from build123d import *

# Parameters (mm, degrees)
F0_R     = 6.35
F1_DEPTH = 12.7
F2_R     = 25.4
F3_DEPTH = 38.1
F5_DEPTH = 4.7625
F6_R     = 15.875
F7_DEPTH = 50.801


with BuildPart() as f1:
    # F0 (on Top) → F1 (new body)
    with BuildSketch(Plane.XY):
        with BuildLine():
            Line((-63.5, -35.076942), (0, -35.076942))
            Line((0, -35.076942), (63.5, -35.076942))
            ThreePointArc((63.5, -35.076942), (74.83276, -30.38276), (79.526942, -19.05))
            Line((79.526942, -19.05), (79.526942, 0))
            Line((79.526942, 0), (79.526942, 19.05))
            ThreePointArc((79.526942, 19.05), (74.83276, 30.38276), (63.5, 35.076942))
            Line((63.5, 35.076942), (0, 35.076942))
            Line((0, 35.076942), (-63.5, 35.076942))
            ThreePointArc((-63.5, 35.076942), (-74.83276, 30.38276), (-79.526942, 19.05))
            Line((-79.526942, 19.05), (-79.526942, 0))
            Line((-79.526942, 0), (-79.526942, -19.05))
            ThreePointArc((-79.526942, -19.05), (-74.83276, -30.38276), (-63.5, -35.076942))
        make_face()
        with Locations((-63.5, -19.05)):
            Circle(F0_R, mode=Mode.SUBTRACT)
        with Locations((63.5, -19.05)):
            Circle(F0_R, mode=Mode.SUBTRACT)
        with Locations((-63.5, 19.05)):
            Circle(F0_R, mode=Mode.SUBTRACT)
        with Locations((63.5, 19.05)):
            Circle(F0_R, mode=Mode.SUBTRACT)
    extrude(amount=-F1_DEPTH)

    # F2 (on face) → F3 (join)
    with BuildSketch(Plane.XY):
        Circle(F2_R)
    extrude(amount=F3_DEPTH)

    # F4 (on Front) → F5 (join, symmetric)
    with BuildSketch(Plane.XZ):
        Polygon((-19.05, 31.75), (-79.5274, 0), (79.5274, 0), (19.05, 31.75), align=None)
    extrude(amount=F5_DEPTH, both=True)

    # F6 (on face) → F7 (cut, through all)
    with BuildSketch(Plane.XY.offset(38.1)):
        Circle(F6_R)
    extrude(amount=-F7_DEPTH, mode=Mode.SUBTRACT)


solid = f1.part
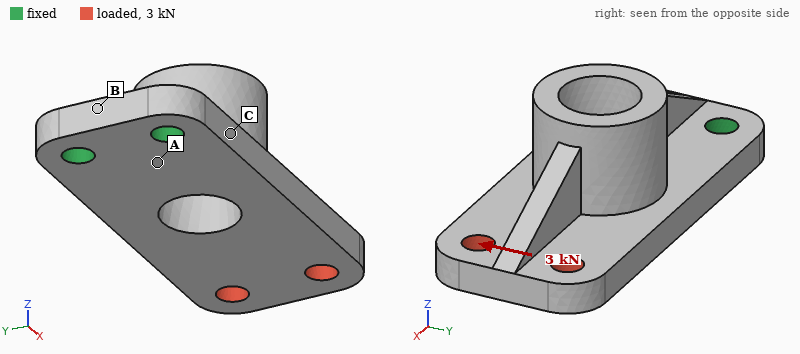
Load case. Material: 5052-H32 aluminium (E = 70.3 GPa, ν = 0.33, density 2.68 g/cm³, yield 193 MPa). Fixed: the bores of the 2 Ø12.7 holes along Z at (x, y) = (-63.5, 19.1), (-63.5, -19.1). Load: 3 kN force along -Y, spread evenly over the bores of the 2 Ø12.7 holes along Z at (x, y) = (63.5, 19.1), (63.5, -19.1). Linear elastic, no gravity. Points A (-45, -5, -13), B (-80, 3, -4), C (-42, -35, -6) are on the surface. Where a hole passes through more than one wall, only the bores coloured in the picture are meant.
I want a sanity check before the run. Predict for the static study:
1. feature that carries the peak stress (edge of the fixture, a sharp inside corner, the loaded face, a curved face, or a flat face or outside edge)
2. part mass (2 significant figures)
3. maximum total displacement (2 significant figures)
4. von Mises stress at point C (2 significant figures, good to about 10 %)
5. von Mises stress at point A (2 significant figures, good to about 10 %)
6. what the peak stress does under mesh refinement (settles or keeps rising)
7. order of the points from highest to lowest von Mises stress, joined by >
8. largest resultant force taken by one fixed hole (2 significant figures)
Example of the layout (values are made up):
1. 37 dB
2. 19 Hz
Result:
1. edge of the fixture
2. 490 g
3. 0.13 mm
4. 28 MPa
5. 14 MPa
6. keeps rising
7. C > A > B
8. 8.3 kN
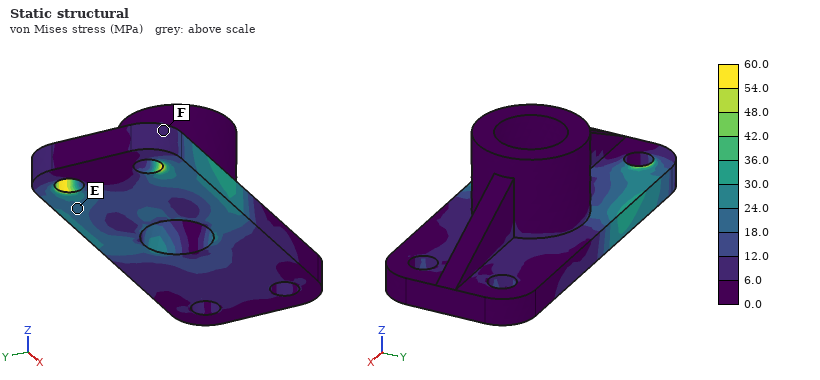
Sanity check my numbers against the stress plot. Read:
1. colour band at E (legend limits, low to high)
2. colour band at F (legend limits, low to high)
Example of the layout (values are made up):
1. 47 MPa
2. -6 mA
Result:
1. 18.0 to 24.0 MPa
2. 6.0 to 12.0 MPa
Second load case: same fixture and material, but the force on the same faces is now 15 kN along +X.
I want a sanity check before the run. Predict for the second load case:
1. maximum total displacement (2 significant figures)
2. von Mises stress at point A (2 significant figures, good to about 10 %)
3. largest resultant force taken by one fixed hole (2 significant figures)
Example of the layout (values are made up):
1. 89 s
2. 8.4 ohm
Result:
1. 0.10 mm
2. 12 MPa
3. 7.5 kN
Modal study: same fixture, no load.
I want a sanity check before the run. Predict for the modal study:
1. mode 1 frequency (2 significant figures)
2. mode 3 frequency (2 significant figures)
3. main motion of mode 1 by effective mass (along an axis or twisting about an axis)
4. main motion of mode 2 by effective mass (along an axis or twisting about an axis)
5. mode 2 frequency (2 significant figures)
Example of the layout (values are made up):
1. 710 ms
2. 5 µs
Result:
1. 760 Hz
2. 2300 Hz
3. along Z
4. along Y
5. 2000 Hz
